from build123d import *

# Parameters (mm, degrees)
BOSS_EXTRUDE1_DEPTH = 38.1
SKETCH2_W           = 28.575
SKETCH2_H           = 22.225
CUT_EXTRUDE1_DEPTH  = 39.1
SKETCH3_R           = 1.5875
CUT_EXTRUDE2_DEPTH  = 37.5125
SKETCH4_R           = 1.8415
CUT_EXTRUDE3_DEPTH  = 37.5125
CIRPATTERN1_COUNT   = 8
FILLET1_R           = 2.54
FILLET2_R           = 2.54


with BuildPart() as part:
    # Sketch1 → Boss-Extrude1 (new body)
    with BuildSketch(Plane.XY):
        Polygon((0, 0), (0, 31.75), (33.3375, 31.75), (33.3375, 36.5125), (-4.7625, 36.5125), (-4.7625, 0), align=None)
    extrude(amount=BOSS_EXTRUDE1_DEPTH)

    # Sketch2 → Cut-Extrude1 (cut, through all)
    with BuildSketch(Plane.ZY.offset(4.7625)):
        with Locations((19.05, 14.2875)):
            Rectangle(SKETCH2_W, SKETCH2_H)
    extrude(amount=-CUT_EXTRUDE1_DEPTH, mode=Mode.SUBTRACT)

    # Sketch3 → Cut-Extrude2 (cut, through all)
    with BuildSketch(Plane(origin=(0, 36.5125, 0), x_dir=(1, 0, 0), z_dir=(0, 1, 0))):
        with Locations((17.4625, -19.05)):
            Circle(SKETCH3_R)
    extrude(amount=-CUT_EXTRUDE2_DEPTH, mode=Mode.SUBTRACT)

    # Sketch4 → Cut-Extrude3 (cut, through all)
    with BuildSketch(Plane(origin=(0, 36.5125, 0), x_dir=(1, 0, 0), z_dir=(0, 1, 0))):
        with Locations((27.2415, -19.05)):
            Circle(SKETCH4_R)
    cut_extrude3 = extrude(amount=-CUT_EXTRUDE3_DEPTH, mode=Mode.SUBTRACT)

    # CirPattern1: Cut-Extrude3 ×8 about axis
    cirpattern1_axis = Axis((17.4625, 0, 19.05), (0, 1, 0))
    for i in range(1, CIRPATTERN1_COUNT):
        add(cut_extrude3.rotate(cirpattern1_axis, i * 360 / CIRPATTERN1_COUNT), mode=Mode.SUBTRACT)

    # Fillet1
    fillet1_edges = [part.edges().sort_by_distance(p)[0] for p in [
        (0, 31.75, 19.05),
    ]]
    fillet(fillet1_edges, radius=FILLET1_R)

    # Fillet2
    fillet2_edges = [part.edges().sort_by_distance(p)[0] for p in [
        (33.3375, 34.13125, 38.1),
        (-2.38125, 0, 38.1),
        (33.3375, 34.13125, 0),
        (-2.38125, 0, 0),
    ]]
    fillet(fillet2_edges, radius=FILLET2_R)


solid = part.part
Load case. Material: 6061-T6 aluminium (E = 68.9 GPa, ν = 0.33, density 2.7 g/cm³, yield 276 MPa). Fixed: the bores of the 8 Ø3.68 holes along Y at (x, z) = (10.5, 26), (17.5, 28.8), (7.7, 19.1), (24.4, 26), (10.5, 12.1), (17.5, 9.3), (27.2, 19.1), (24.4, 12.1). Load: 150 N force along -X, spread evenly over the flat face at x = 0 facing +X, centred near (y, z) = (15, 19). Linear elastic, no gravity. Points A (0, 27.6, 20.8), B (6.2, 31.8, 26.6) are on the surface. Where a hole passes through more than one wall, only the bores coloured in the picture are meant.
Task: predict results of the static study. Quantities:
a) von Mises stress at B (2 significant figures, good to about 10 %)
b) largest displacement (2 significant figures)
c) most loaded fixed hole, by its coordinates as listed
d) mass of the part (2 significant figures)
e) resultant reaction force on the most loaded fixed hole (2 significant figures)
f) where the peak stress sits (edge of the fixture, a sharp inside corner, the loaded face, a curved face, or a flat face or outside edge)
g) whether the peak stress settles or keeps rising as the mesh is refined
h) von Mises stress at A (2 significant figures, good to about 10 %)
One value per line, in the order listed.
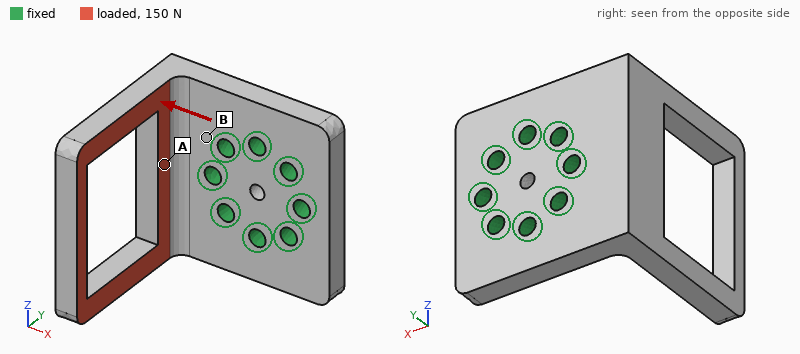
18 MPa
0.14 mm
(7.7, 19.1)
25 g
130 N
edge of the fixture
keeps rising
6.2 MPa
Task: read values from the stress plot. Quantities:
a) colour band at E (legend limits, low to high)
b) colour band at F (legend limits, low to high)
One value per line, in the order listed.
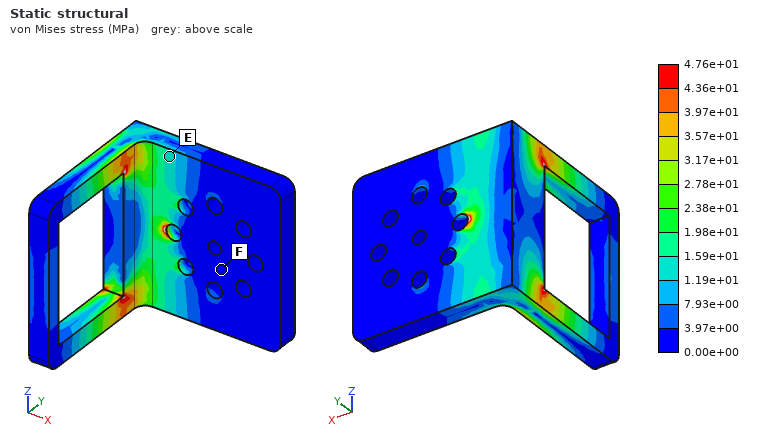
1.19e+01 to 1.59e+01 MPa
0.00e+00 to 3.97e+00 MPa
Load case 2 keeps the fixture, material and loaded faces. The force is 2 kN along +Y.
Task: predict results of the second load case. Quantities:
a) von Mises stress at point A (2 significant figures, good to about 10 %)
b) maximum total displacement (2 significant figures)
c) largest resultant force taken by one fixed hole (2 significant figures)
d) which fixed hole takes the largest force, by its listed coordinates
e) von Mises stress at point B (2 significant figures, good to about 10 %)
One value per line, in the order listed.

39 MPa
0.19 mm
1.0 kN
(7.7, 19.1)
82 MPa
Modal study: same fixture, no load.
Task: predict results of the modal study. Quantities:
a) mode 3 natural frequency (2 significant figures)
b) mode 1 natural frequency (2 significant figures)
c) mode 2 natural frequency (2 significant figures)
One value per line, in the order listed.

4700 Hz
2500 Hz
3600 Hz
